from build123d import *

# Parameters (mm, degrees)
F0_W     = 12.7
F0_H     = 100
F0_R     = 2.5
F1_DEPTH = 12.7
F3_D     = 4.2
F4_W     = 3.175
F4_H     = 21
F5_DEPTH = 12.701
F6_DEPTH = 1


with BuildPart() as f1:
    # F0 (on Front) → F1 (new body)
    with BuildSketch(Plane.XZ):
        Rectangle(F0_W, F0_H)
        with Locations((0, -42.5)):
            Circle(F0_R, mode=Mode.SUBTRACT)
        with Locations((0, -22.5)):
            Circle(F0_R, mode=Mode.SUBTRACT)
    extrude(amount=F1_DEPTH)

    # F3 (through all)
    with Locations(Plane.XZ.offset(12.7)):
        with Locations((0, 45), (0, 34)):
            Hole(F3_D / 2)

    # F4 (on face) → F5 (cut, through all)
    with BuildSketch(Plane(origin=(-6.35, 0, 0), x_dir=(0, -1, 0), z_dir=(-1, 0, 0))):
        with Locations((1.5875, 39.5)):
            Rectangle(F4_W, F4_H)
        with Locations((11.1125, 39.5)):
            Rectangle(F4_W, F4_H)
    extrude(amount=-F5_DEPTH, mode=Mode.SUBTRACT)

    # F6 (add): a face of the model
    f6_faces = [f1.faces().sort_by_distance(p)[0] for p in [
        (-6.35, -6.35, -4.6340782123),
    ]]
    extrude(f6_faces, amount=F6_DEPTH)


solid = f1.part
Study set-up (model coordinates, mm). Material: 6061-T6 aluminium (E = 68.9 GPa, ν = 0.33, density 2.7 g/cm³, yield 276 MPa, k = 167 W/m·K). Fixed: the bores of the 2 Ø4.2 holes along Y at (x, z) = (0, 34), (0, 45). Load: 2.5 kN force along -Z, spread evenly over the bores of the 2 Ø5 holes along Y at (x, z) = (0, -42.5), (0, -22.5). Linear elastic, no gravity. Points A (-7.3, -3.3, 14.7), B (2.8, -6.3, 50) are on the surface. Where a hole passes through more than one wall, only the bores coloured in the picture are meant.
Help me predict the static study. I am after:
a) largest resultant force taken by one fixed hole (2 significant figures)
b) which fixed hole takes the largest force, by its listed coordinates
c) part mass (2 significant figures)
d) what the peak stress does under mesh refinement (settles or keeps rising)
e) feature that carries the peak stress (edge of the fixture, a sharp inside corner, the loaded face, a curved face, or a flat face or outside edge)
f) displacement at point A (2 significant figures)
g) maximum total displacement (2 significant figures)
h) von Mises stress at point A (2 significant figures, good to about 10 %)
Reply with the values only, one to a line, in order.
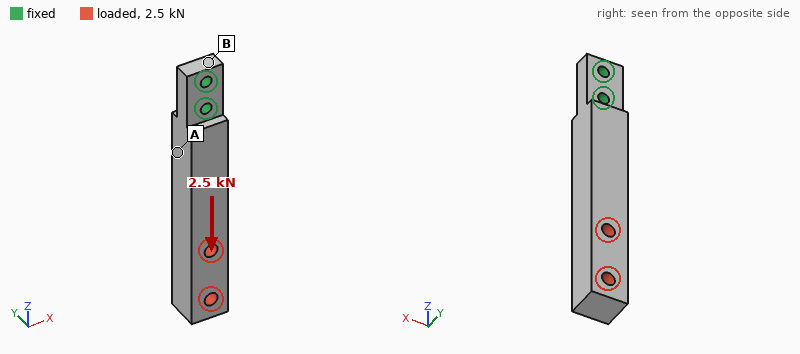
2.2 kN
(0, 34)
40 g
keeps rising
edge of the fixture
5.0 µm
32 µm
11 MPa
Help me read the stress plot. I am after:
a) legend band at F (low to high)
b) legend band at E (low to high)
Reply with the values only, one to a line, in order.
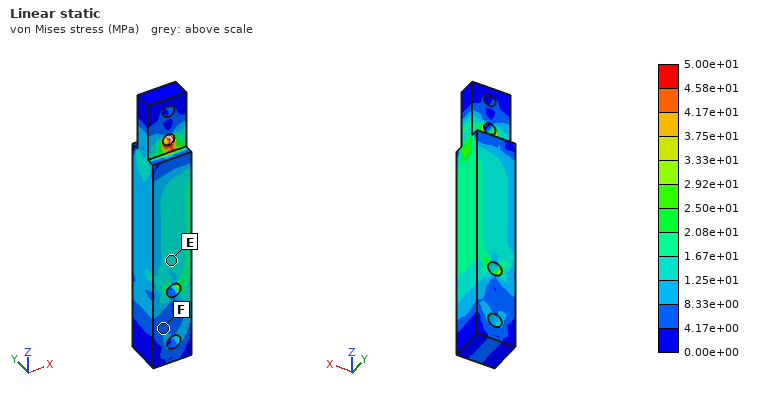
4.17e+00 to 8.33e+00 MPa
1.25e+01 to 1.67e+01 MPa
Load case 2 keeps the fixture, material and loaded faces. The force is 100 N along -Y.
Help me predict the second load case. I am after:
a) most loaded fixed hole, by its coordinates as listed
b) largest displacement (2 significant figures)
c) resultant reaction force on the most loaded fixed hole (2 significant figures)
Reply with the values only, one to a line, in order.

(0, 34)
0.22 mm
220 N
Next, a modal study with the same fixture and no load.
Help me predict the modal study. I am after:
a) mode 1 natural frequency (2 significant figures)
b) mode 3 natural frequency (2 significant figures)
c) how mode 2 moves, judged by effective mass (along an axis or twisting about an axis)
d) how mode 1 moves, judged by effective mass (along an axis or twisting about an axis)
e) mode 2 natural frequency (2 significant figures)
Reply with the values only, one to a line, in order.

900 Hz
6900 Hz
along X
along Y
1200 Hz
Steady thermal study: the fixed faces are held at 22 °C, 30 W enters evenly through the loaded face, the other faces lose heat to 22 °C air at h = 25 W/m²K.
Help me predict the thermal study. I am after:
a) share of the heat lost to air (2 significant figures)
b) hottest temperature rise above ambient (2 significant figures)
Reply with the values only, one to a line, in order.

16 %
68 K
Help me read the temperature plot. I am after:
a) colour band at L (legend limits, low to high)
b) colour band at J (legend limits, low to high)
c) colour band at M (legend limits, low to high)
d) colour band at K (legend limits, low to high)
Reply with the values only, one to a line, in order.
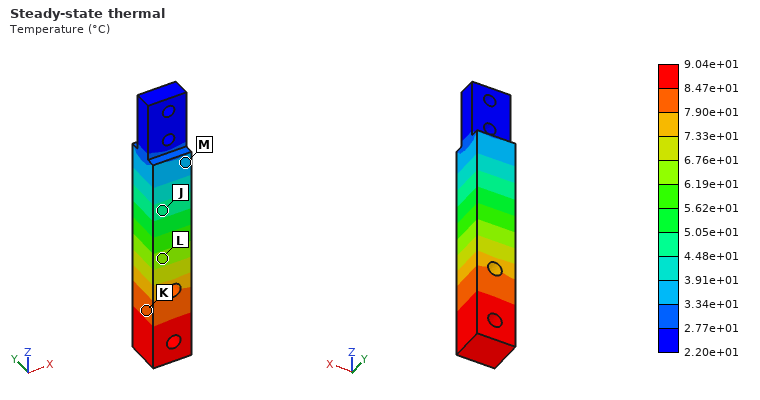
6.19e+01 to 6.76e+01 °C
4.48e+01 to 5.05e+01 °C
3.34e+01 to 3.91e+01 °C
7.90e+01 to 8.47e+01 °C
